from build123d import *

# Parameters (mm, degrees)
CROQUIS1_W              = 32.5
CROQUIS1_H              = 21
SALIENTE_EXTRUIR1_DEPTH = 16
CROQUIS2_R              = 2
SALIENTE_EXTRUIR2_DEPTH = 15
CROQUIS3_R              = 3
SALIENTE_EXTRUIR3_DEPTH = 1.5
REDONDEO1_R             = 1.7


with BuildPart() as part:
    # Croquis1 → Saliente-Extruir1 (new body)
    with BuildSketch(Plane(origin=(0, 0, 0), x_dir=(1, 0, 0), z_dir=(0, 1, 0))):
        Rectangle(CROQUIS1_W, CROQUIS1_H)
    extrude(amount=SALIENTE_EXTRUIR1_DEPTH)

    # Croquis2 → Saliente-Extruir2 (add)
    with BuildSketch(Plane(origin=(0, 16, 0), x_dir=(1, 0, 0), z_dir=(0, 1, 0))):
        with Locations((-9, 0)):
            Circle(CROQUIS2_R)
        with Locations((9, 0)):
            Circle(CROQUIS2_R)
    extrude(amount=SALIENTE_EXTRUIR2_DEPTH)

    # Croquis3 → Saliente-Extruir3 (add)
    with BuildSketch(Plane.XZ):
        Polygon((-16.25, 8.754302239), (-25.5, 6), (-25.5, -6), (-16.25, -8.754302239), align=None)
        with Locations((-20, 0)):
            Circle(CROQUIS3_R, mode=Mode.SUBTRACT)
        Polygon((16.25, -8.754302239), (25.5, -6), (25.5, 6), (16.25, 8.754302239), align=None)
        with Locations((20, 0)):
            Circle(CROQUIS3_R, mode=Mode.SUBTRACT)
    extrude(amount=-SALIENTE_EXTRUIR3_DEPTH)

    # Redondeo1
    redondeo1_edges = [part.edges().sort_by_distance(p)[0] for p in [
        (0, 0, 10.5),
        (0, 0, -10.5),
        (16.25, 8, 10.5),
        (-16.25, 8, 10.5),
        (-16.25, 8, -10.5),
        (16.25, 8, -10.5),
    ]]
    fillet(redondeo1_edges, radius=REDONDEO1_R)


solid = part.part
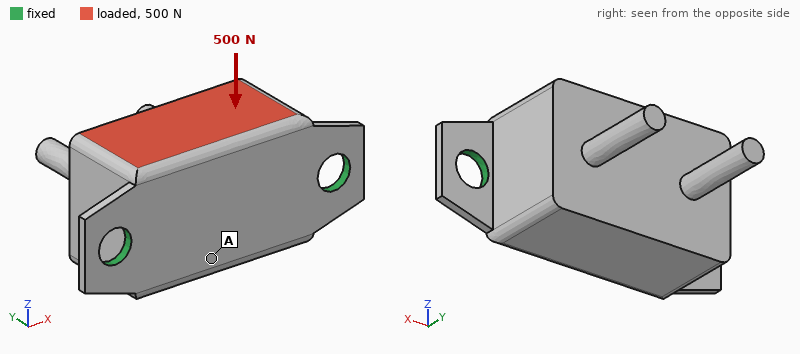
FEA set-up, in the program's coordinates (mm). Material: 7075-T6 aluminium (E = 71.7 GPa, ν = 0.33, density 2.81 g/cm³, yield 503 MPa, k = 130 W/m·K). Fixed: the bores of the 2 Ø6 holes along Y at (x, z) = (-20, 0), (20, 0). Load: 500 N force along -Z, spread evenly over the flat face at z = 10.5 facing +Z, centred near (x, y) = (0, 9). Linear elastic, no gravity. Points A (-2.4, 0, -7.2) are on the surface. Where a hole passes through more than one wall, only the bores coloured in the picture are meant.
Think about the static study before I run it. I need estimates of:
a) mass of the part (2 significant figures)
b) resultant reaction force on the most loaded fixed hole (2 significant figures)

32 g
250 N
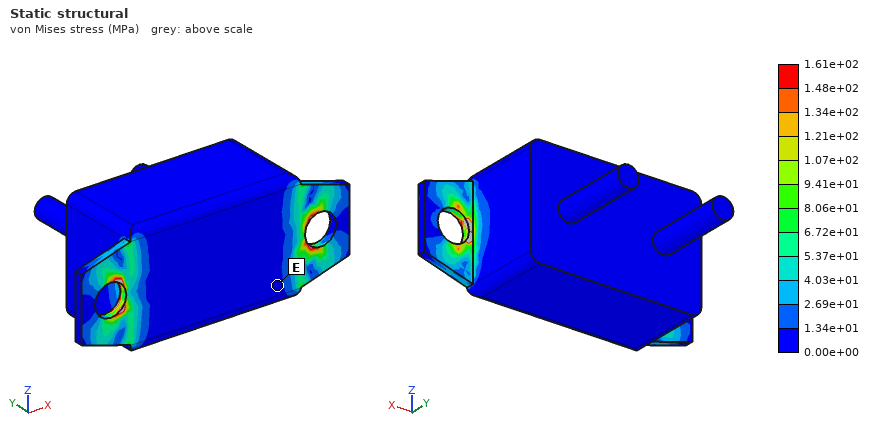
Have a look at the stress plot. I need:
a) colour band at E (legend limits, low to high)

0.00e+00 to 1.34e+01 MPa
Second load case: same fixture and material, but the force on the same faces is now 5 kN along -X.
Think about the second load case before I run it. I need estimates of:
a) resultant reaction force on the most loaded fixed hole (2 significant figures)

3.1 kN
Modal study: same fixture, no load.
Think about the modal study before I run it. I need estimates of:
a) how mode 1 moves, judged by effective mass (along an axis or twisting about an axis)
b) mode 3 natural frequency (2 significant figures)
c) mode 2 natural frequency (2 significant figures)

along Z
11 kHz
10 kHz
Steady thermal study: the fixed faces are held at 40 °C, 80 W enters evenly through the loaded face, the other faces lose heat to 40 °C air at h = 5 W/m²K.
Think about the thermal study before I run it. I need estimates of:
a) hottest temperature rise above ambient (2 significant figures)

73 K
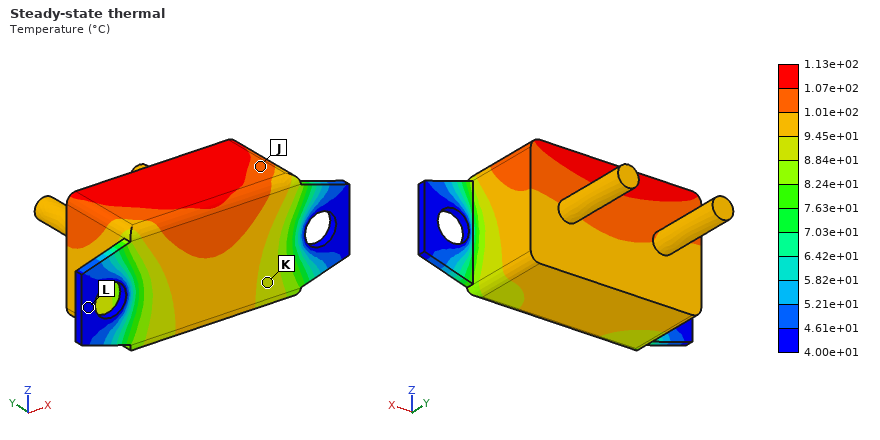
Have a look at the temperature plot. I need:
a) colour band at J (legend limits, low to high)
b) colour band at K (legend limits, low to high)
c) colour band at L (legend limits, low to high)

1.01e+02 to 1.07e+02 °C
8.84e+01 to 9.45e+01 °C
4.00e+01 to 4.61e+01 °C
